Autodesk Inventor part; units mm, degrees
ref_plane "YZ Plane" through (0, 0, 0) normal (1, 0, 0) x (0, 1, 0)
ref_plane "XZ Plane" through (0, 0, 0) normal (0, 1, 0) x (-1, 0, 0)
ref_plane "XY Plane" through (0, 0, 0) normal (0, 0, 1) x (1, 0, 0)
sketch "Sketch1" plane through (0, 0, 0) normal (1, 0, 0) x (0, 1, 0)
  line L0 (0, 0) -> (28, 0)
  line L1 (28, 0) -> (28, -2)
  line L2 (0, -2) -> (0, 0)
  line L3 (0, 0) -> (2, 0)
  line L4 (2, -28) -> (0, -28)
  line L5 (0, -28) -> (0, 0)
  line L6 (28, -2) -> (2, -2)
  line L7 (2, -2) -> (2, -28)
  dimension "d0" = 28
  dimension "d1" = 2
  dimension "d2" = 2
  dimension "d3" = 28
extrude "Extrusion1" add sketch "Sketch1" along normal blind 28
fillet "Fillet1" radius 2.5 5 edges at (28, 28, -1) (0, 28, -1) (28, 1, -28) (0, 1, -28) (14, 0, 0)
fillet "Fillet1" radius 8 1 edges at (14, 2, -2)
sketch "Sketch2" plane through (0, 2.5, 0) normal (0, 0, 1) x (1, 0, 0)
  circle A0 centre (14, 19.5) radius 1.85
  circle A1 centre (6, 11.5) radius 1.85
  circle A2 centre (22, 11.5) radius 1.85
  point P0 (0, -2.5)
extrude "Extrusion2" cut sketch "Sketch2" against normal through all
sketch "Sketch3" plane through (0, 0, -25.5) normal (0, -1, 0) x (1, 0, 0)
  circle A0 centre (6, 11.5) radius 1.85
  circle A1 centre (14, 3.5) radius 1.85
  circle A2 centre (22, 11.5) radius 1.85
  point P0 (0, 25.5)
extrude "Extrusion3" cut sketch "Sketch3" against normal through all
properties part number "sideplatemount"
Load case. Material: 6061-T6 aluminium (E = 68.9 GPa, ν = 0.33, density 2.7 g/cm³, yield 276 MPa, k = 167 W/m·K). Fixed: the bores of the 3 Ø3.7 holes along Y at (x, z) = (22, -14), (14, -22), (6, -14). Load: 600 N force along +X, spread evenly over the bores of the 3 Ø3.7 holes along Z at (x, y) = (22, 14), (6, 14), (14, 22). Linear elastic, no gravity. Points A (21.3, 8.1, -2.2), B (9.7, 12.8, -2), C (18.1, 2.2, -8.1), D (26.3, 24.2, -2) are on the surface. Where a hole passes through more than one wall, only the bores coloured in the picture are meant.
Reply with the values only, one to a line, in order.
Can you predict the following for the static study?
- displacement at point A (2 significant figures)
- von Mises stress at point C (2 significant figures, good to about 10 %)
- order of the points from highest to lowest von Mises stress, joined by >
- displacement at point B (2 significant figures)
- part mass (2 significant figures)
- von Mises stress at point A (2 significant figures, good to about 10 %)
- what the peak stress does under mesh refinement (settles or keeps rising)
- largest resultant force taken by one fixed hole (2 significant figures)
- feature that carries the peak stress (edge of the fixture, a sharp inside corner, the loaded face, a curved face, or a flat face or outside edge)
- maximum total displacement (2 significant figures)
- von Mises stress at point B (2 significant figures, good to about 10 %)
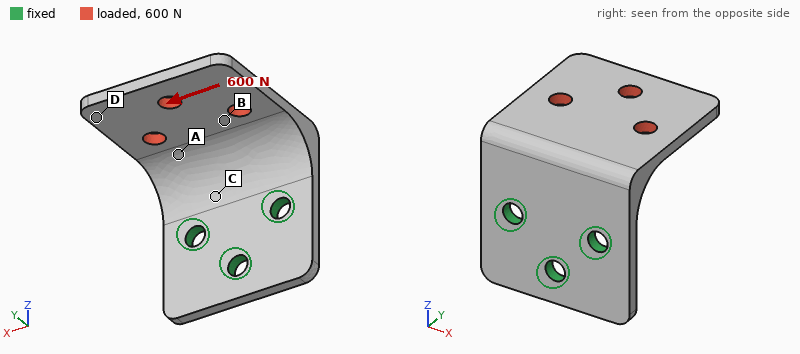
0.085 mm
120 MPa
C > A > B > D
0.11 mm
8.7 g
72 MPa
keeps rising
720 N
edge of the fixture
0.26 mm
43 MPa
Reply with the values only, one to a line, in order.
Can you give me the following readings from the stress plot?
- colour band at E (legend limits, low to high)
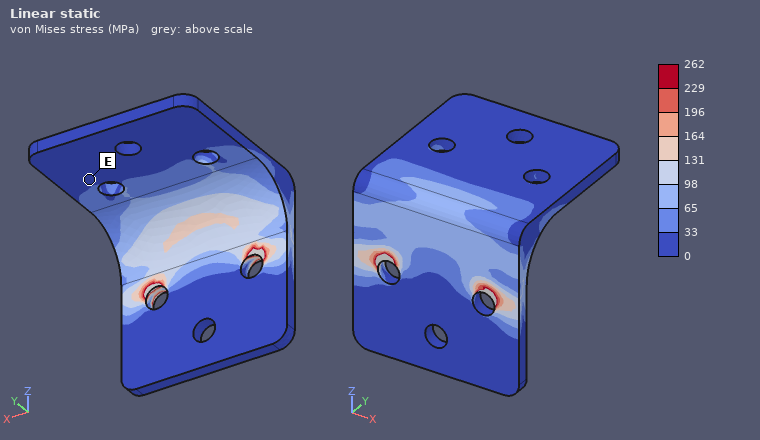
0 to 33 MPa
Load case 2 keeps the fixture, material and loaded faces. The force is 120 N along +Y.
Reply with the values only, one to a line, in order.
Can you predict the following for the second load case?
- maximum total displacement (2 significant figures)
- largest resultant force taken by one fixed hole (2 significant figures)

0.15 mm
73 N
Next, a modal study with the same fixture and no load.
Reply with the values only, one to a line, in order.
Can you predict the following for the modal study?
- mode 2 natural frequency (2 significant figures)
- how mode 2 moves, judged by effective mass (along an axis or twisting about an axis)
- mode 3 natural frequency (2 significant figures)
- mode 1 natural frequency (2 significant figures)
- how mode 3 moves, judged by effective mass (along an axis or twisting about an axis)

4400 Hz
along X
5900 Hz
1800 Hz
along Y
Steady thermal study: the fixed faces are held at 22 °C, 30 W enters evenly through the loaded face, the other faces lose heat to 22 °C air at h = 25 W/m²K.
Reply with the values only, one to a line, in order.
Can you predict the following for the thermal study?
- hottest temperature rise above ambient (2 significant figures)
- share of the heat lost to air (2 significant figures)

74 K
7.9 %
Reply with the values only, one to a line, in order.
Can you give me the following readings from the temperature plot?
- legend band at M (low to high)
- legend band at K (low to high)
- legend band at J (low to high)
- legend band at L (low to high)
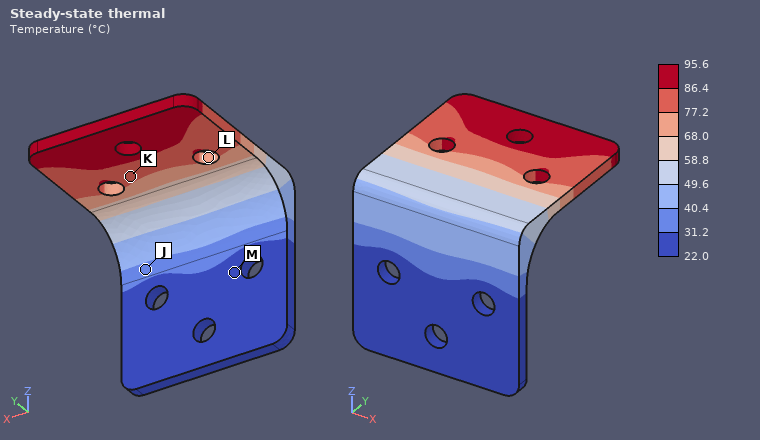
22.0 to 31.2 °C
77.2 to 86.4 °C
31.2 to 40.4 °C
68.0 to 77.2 °C
